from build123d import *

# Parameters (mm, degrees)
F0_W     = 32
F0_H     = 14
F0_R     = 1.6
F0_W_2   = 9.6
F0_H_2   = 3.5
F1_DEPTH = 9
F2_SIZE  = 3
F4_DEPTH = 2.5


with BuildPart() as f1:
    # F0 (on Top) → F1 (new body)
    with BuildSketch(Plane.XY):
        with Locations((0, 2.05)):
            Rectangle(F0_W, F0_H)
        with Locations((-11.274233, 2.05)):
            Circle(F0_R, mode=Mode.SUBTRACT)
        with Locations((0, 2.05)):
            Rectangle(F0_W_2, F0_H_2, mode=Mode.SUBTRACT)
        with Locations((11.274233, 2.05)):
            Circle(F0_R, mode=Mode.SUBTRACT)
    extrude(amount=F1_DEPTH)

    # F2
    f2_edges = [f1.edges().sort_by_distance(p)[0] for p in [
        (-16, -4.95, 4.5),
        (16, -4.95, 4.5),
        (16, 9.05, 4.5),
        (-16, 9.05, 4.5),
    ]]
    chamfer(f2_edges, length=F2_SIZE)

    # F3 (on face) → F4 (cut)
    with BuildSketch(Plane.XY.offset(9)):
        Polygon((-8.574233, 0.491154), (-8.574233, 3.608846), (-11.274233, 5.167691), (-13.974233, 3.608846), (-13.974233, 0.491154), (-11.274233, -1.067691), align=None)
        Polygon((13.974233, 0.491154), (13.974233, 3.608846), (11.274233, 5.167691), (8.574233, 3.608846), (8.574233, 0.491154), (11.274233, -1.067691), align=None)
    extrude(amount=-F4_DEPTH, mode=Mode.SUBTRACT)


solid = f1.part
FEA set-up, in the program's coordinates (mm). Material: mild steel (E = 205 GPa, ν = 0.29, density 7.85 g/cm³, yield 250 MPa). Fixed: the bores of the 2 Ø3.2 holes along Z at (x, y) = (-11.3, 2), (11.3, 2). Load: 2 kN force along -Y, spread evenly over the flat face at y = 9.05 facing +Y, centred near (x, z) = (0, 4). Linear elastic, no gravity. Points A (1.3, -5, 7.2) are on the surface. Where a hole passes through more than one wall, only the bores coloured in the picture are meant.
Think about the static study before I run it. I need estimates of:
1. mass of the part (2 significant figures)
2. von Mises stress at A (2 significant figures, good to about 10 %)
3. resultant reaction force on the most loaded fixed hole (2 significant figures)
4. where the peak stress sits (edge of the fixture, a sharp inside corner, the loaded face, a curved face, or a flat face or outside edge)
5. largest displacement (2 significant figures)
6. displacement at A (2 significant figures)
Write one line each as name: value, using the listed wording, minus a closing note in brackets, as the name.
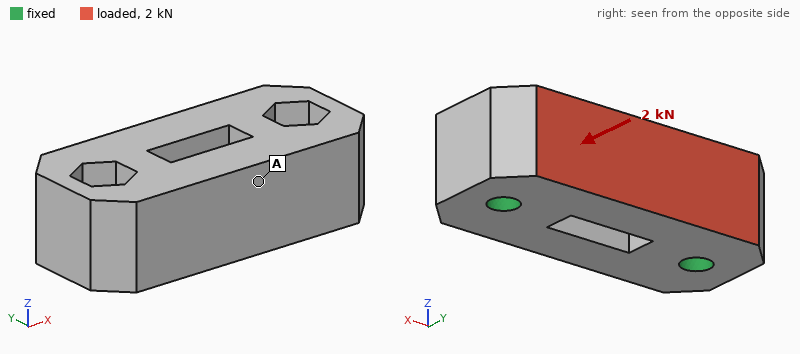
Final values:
mass of the part: 26 g
von Mises stress at A: 7.5 MPa
resultant reaction force on the most loaded fixed hole: 1.0 kN
where the peak stress sits: edge of the fixture
largest displacement: 2.2 µm
displacement at A: 0.92 µm
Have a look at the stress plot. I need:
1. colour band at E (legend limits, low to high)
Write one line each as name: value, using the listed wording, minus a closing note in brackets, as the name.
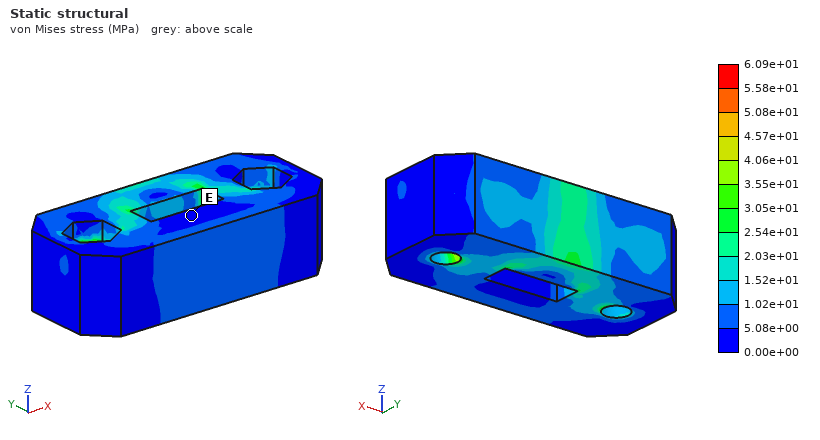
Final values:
colour band at E: 0.00e+00 to 5.08e+00 MPa
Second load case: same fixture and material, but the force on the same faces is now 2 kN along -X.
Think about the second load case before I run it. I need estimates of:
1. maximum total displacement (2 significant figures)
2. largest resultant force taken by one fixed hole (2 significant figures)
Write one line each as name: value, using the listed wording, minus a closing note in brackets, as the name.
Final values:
maximum total displacement: 1.5 µm
largest resultant force taken by one fixed hole: 1.1 kN
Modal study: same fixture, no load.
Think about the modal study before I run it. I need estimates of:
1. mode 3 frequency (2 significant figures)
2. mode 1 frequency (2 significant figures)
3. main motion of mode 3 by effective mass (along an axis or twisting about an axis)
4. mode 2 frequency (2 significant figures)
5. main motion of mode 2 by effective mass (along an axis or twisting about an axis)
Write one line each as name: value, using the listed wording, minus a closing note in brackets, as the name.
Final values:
mode 3 frequency: 52 kHz
mode 1 frequency: 40 kHz
main motion of mode 3 by effective mass: along Y
mode 2 frequency: 44 kHz
main motion of mode 2 by effective mass: along Z
